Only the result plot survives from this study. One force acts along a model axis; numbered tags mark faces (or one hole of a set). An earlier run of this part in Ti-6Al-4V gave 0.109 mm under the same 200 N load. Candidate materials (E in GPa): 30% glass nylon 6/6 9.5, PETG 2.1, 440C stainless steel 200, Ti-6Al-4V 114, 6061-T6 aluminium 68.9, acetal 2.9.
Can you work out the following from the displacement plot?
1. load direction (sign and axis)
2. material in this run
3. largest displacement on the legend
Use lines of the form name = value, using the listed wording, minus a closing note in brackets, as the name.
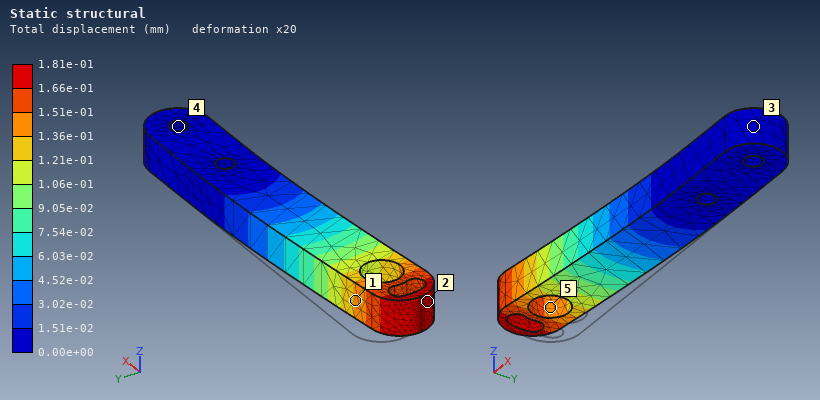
load direction = -Y
material in this run = 6061-T6 aluminium
largest displacement on the legend = 1.81e-01 mm
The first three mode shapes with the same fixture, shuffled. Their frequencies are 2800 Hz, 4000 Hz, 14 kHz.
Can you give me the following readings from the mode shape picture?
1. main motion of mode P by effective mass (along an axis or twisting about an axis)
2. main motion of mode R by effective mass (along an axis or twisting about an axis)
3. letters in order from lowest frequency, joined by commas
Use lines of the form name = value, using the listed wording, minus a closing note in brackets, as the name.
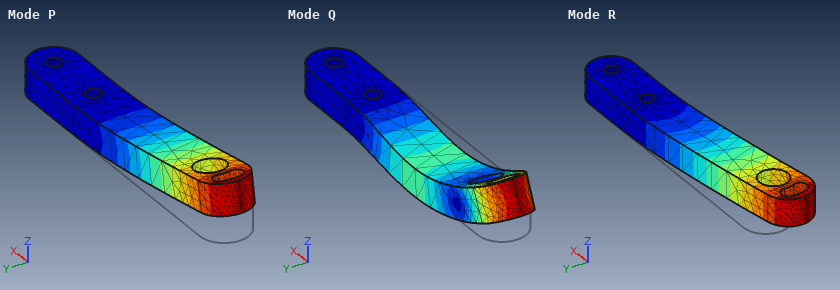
main motion of mode P by effective mass = along Z
main motion of mode R by effective mass = along Y
letters in order from lowest frequency, joined by commas = P, R, Q
